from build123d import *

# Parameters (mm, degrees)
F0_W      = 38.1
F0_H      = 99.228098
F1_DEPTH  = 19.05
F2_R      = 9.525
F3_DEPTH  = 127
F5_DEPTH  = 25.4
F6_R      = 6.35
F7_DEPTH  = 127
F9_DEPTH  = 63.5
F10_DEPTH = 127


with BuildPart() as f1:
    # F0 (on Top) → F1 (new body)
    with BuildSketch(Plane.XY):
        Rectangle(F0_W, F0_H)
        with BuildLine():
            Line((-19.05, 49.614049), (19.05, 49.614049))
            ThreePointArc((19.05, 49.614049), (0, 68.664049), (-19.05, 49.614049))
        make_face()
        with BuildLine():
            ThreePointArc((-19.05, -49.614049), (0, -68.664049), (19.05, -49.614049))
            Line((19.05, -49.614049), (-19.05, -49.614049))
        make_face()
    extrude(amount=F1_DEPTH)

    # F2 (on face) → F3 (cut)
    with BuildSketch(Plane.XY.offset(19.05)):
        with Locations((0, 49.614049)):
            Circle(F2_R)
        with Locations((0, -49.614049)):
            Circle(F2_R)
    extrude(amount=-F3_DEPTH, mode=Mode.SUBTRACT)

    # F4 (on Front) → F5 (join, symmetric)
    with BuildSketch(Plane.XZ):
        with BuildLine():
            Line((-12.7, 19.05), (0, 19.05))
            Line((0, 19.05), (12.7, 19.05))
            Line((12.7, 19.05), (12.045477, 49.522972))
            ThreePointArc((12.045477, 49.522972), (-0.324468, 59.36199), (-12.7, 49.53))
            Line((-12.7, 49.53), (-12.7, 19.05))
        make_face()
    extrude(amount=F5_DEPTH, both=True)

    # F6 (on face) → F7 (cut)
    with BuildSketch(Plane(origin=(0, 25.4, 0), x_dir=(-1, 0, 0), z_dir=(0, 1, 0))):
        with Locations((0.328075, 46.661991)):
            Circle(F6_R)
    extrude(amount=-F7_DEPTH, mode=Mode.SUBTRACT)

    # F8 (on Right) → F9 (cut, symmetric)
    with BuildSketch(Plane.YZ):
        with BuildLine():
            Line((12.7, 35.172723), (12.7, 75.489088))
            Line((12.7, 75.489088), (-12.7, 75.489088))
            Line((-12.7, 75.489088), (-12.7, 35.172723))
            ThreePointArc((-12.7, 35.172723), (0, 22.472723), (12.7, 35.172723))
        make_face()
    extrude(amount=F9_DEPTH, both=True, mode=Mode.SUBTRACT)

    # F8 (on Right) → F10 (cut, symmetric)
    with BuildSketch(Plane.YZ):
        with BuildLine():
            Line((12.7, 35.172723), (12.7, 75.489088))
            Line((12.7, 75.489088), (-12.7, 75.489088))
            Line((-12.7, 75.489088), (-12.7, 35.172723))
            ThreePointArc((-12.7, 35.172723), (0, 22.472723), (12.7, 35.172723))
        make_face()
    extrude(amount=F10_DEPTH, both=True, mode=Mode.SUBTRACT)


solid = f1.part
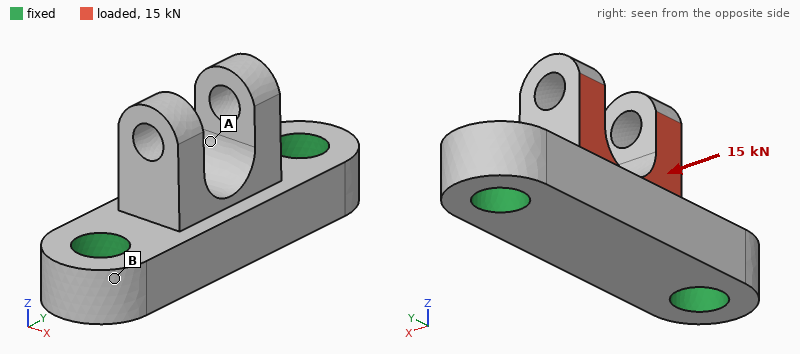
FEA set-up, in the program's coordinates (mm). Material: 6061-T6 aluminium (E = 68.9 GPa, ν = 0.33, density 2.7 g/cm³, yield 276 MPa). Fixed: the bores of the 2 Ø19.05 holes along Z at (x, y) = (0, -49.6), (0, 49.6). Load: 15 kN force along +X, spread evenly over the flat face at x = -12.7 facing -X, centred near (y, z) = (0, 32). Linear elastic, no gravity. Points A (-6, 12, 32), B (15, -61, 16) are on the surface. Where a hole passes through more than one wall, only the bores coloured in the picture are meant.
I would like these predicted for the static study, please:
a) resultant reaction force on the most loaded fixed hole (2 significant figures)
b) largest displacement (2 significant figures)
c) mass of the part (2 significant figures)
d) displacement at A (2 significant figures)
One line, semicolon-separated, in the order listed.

7.5 kN; 0.18 mm; 290 g; 0.083 mm
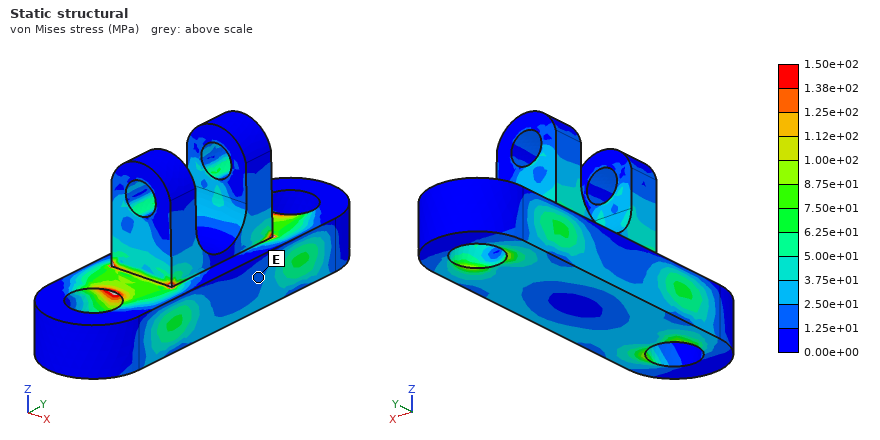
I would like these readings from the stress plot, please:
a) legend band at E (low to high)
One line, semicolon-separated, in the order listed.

1.25e+01 to 2.50e+01 MPa
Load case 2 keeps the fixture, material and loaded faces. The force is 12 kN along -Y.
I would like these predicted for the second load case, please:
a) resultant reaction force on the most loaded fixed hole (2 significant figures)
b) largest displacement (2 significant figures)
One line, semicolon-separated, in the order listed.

7.3 kN; 97 µm
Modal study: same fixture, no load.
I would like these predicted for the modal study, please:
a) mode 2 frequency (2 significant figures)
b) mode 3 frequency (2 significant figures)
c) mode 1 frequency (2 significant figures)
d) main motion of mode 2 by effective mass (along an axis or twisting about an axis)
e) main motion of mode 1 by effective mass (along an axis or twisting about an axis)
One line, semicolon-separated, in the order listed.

7500 Hz; 8200 Hz; 6200 Hz; along Z; along X
